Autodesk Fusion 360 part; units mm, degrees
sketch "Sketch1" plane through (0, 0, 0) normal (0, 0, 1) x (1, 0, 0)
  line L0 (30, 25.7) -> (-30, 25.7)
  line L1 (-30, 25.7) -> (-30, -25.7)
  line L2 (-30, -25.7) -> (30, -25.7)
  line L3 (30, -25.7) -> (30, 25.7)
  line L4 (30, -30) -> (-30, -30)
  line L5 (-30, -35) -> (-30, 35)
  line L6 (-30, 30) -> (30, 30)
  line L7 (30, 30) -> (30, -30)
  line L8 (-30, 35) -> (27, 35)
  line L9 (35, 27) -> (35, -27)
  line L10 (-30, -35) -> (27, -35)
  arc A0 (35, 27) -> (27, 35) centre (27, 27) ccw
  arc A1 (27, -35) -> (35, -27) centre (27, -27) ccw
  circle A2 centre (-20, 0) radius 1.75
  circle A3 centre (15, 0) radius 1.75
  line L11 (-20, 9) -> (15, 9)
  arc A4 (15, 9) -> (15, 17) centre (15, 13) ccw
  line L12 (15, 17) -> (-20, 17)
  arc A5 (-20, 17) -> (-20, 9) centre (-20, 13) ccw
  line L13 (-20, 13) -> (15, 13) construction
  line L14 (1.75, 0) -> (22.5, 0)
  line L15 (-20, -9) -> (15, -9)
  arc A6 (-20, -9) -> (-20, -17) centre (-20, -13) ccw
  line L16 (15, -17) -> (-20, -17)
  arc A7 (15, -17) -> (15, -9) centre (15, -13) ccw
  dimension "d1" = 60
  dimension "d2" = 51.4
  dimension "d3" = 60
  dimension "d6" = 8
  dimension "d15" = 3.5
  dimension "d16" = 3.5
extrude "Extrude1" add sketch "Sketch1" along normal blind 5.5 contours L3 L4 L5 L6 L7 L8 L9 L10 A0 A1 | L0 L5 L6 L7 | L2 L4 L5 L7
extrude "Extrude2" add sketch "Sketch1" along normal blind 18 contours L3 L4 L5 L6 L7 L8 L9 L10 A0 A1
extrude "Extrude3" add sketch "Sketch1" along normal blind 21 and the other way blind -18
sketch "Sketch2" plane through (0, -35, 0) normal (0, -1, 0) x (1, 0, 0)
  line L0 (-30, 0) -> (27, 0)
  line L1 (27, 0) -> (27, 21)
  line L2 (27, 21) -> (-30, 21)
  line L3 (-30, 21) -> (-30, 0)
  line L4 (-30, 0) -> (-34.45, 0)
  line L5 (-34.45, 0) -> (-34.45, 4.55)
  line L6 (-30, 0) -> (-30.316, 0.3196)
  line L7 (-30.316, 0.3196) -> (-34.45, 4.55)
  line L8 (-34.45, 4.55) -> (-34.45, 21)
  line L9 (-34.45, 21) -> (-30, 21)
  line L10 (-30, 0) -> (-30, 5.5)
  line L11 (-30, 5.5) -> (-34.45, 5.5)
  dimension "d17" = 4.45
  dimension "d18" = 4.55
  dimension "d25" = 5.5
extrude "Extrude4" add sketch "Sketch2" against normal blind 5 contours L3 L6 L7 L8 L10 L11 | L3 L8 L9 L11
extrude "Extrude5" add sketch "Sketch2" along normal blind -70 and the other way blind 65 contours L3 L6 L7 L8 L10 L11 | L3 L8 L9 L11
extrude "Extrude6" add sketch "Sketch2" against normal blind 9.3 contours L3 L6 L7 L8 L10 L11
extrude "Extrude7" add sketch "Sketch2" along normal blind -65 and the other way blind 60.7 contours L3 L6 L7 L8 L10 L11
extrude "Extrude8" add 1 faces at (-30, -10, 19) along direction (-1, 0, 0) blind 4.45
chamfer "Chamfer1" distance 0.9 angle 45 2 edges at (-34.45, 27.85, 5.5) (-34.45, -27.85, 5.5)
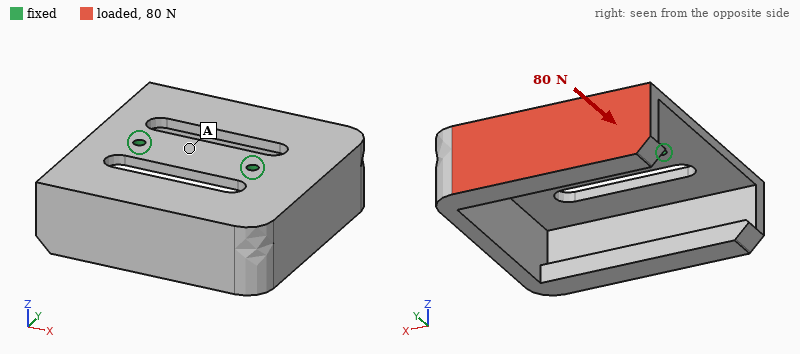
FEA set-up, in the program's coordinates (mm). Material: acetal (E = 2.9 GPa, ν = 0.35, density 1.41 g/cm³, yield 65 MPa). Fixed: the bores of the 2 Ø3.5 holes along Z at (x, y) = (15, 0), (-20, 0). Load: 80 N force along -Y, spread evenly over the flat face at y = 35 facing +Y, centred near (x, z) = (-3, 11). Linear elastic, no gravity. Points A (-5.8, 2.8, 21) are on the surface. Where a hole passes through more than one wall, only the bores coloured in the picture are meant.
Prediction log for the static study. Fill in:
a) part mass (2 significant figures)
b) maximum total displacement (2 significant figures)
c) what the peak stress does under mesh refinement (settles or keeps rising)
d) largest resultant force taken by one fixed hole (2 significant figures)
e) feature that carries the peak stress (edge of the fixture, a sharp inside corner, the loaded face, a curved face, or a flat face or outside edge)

46 g
1.1 mm
keeps rising
43 N
edge of the fixture
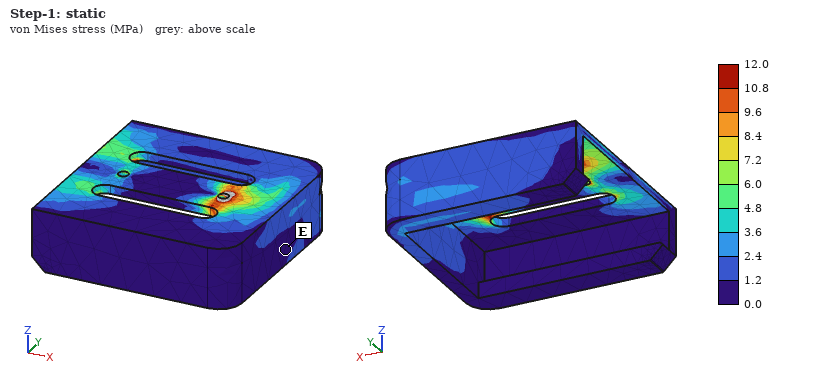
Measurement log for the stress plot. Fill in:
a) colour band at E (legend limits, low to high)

0.0 to 1.2 MPa
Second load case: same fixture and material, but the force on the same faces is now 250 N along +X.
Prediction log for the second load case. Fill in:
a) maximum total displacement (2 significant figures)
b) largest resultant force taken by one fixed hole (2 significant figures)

1.1 mm
270 N
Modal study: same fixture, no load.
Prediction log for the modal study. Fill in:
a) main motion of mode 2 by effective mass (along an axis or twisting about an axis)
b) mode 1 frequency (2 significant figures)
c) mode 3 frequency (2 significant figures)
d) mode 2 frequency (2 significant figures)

along Z
160 Hz
520 Hz
360 Hz
